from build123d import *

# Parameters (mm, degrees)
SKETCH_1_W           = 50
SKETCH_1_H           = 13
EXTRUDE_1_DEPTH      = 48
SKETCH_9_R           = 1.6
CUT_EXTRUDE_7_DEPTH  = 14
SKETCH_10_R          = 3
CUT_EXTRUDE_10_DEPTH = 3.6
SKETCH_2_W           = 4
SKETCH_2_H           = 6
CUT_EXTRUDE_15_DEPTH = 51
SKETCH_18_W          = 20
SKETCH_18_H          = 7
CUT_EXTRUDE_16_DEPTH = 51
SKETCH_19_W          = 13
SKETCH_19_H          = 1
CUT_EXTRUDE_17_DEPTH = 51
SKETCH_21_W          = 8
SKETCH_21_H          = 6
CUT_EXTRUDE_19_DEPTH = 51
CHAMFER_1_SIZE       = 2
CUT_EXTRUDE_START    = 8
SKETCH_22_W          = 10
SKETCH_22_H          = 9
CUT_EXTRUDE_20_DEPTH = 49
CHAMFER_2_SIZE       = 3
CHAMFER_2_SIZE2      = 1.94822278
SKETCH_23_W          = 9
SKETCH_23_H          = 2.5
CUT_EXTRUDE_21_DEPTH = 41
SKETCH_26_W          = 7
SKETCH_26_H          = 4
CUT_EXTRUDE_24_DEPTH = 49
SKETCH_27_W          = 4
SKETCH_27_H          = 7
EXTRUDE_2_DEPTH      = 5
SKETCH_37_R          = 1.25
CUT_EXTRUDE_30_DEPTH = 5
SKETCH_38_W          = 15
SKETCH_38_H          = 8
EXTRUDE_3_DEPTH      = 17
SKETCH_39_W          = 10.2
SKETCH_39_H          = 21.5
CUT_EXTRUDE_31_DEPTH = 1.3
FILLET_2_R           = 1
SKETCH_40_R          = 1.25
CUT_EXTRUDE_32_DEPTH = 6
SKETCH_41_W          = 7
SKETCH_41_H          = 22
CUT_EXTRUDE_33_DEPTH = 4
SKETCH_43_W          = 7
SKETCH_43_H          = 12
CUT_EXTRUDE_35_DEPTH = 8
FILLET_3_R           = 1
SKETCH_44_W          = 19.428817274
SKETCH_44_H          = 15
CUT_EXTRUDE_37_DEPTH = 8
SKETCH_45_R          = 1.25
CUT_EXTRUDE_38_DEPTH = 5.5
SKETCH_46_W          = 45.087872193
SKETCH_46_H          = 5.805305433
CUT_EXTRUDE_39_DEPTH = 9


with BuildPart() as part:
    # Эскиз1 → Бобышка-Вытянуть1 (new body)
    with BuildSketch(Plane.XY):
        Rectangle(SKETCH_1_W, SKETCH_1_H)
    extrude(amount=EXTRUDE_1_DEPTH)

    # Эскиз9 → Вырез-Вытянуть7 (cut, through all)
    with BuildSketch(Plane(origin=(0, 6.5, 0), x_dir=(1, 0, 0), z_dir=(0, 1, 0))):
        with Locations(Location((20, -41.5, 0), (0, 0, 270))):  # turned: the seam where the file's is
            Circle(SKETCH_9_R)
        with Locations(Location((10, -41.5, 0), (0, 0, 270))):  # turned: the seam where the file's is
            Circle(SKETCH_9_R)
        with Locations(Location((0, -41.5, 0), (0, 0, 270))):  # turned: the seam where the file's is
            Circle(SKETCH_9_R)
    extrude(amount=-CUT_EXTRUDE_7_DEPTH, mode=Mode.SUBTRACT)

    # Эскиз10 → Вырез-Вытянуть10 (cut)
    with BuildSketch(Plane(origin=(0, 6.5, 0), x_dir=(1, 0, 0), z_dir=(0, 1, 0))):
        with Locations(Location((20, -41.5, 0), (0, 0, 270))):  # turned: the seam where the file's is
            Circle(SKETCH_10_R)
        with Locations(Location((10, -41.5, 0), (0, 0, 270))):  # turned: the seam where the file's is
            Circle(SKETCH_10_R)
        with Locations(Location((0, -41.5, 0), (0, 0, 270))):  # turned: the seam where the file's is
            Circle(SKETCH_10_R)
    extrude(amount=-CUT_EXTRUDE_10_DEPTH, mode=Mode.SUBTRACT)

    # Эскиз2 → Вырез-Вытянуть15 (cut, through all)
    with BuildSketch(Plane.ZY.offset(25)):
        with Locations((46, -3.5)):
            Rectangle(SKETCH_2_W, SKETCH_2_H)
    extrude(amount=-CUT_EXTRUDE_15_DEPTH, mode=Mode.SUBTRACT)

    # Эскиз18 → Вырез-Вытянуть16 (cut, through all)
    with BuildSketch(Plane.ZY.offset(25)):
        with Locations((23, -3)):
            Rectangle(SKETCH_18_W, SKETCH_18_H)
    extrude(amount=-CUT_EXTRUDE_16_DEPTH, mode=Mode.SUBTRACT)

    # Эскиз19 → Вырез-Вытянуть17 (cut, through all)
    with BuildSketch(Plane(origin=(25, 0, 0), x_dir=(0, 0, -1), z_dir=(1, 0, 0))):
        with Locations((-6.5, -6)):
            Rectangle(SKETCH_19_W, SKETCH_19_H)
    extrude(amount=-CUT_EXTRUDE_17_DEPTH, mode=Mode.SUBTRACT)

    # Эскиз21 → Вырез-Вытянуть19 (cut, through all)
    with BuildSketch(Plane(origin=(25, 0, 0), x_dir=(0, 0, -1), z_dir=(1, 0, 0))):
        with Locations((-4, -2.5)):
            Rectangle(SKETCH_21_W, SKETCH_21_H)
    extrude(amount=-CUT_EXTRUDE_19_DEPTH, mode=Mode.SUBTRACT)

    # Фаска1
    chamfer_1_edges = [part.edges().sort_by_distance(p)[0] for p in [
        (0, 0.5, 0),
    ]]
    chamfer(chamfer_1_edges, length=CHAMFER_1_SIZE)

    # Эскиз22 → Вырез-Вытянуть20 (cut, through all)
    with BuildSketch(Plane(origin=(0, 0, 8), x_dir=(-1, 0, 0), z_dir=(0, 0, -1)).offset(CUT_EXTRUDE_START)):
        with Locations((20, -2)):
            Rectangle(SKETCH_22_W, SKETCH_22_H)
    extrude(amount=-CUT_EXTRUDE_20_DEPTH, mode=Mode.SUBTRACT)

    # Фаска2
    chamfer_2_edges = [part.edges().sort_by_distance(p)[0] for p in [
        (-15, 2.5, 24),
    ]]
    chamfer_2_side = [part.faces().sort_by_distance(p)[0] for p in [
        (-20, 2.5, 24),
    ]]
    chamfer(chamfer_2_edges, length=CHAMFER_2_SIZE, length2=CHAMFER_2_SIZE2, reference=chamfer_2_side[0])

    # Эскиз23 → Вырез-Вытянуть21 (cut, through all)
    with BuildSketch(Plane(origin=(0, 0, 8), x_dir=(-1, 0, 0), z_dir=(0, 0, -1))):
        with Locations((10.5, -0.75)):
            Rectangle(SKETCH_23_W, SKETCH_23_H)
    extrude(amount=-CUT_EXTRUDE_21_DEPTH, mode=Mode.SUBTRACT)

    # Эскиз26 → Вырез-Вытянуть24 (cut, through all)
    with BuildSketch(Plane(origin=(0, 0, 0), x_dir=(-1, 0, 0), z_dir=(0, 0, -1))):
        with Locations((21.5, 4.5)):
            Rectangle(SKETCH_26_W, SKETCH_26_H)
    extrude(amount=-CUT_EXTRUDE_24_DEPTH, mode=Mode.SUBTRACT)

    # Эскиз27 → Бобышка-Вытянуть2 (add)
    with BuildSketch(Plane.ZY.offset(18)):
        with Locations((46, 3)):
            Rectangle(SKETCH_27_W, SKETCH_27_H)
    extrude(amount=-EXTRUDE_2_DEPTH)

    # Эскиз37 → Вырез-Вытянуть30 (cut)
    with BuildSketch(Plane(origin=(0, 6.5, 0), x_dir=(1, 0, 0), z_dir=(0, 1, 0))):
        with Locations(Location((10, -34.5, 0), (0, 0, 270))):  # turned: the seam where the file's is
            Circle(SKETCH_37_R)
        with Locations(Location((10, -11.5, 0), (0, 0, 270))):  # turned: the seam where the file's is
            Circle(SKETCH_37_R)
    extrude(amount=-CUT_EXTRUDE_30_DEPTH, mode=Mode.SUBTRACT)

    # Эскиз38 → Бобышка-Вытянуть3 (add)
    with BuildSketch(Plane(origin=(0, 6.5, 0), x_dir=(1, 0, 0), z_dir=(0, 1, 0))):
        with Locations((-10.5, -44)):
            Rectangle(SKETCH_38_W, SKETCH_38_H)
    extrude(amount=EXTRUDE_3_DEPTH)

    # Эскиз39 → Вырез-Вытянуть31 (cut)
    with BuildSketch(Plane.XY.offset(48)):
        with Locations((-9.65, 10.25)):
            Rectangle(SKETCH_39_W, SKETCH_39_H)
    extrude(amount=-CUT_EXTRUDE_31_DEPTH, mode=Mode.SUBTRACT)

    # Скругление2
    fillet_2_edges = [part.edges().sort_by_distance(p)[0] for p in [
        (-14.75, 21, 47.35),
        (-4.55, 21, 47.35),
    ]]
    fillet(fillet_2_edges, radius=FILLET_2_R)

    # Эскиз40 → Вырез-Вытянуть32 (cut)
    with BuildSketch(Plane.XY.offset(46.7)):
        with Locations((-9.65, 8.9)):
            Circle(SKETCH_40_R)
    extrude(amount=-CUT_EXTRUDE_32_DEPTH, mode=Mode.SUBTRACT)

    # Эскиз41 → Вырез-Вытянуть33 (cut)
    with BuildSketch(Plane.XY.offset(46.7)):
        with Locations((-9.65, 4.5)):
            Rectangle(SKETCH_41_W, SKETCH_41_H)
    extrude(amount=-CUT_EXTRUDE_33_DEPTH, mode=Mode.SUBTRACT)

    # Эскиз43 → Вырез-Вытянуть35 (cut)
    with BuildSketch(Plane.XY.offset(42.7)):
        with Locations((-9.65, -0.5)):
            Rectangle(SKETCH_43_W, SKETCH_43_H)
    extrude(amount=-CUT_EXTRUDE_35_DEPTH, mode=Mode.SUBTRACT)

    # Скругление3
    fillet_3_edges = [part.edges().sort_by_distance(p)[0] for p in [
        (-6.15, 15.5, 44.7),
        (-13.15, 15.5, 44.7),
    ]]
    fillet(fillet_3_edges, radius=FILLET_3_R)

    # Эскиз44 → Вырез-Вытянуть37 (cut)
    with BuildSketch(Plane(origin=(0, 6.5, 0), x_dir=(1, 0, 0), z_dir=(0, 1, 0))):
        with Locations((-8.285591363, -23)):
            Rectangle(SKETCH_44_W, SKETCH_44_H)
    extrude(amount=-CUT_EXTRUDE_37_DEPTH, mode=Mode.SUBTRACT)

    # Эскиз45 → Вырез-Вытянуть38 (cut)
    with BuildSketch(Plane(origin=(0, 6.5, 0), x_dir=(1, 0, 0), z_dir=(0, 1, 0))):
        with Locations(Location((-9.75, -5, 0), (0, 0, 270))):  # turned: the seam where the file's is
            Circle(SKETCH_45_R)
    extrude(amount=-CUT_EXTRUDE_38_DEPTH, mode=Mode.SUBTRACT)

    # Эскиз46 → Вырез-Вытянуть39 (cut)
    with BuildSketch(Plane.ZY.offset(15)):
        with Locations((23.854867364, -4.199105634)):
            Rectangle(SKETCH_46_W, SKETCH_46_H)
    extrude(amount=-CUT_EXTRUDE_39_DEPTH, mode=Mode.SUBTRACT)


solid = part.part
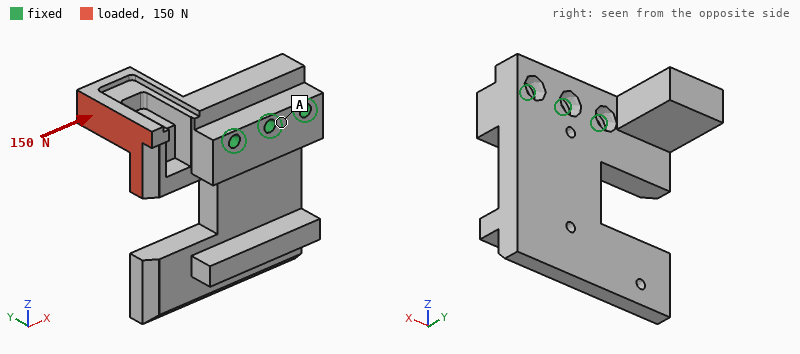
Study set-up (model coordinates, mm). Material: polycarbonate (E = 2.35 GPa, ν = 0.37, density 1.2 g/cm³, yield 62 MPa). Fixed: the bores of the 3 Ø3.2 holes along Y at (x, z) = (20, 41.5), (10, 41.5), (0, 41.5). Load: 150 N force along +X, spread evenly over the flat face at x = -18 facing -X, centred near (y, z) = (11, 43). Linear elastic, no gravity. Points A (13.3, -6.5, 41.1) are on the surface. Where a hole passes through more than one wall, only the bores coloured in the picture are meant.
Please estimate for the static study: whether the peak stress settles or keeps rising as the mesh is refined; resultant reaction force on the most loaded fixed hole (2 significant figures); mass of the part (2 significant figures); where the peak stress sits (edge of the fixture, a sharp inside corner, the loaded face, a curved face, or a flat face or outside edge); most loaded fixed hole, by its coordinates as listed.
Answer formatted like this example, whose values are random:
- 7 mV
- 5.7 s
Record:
- keeps rising
- 100 N
- 17 g
- a sharp inside corner
- (0, 41.5)
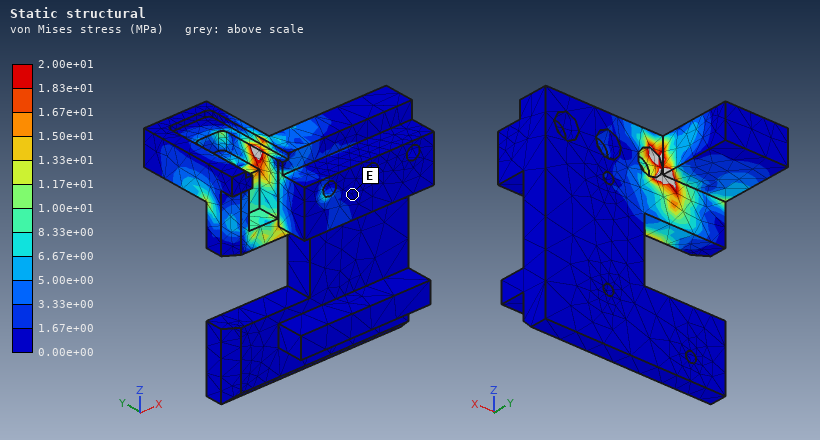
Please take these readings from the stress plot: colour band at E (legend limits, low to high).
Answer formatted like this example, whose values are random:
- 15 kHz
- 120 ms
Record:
- 0.00e+00 to 1.67e+00 MPa
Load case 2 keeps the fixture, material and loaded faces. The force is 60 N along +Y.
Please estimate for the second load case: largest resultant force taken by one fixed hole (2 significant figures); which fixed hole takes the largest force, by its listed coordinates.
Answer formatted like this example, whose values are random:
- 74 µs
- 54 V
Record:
- 110 N
- (0, 41.5)
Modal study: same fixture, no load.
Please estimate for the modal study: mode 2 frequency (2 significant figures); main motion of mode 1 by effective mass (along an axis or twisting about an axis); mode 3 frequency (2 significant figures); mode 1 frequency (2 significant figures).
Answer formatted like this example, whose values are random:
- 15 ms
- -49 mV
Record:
- 1100 Hz
- along Y
- 1400 Hz
- 670 Hz
